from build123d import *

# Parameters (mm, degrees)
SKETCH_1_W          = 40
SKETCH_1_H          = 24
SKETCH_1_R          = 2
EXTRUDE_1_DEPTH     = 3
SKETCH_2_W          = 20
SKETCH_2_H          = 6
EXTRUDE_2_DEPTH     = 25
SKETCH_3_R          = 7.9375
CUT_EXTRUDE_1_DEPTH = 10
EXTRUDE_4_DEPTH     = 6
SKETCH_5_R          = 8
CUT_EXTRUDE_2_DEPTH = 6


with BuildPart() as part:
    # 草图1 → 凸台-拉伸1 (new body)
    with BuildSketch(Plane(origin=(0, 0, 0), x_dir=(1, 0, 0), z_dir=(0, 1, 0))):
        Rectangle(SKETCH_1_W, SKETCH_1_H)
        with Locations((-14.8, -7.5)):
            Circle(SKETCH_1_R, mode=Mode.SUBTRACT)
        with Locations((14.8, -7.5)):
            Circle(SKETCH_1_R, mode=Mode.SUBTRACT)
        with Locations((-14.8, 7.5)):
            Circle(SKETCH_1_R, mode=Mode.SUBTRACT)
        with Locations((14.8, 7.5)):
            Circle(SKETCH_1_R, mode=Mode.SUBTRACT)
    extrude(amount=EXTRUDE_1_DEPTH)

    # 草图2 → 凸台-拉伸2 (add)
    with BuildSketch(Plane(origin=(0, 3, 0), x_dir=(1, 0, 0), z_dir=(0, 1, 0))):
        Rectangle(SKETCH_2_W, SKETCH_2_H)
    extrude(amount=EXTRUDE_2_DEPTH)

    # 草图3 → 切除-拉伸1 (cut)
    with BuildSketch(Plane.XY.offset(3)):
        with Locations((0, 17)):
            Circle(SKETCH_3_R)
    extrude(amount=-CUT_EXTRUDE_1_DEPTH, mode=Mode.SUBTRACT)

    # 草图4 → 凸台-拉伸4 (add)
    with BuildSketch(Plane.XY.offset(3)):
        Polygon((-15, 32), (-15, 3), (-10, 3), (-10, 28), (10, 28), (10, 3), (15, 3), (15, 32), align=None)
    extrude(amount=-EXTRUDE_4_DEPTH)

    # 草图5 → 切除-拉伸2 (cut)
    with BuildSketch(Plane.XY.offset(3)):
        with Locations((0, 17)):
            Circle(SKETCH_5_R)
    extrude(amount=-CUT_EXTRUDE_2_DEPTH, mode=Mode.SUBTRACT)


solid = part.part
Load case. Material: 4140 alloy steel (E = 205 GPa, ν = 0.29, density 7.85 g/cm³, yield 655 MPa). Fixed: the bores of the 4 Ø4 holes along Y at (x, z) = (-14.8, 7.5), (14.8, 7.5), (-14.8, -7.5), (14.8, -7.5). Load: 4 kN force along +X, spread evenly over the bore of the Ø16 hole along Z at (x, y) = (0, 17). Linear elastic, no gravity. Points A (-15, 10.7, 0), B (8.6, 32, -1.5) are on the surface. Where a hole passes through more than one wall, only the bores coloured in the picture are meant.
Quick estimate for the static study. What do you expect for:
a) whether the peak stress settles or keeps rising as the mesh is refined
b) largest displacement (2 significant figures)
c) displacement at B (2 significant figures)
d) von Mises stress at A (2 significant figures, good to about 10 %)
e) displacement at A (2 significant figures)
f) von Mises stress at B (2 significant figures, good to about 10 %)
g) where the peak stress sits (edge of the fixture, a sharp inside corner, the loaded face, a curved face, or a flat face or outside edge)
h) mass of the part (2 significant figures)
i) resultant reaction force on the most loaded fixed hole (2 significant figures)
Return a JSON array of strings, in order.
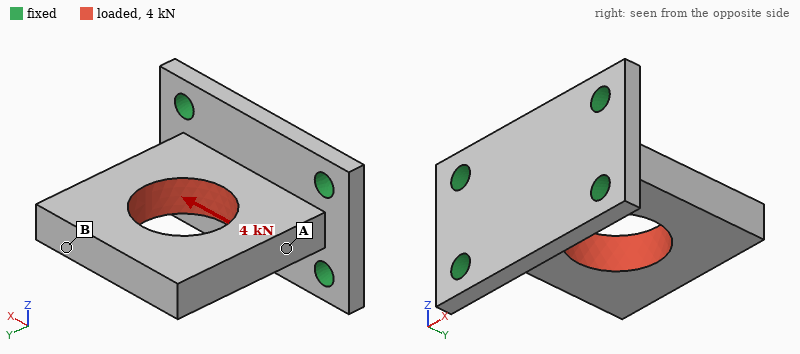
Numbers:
["keeps rising", "35 µm", "34 µm", "87 MPa", "13 µm", "33 MPa", "edge of the fixture", "53 g", "1.5 kN"]
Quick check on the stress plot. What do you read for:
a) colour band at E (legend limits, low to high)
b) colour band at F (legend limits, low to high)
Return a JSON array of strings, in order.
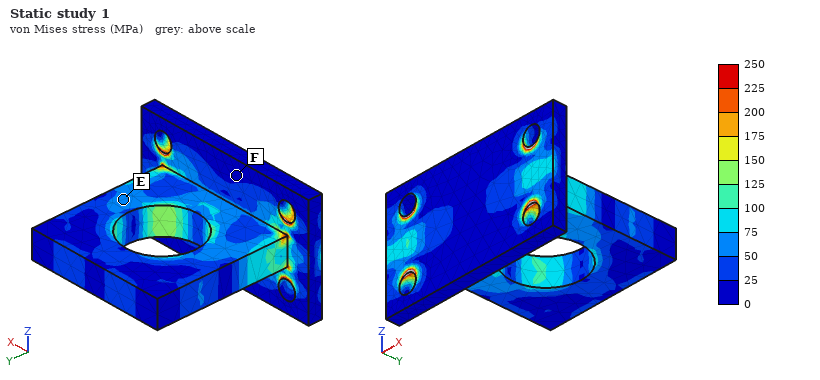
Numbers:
["50 to 75 MPa", "0 to 25 MPa"]
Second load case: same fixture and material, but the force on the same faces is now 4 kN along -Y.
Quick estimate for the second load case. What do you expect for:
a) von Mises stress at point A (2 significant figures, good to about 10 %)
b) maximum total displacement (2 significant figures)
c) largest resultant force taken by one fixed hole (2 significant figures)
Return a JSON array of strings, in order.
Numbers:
["43 MPa", "9.7 µm", "1.1 kN"]
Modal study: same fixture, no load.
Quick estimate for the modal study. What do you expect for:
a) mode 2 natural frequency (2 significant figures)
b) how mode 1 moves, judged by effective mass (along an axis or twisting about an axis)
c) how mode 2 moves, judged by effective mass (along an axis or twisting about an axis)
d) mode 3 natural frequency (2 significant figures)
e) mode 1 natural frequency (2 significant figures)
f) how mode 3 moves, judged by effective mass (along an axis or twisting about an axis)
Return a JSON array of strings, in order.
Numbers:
["9400 Hz", "along Z", "twisting about Y", "10 kHz", "4000 Hz", "along X"]
